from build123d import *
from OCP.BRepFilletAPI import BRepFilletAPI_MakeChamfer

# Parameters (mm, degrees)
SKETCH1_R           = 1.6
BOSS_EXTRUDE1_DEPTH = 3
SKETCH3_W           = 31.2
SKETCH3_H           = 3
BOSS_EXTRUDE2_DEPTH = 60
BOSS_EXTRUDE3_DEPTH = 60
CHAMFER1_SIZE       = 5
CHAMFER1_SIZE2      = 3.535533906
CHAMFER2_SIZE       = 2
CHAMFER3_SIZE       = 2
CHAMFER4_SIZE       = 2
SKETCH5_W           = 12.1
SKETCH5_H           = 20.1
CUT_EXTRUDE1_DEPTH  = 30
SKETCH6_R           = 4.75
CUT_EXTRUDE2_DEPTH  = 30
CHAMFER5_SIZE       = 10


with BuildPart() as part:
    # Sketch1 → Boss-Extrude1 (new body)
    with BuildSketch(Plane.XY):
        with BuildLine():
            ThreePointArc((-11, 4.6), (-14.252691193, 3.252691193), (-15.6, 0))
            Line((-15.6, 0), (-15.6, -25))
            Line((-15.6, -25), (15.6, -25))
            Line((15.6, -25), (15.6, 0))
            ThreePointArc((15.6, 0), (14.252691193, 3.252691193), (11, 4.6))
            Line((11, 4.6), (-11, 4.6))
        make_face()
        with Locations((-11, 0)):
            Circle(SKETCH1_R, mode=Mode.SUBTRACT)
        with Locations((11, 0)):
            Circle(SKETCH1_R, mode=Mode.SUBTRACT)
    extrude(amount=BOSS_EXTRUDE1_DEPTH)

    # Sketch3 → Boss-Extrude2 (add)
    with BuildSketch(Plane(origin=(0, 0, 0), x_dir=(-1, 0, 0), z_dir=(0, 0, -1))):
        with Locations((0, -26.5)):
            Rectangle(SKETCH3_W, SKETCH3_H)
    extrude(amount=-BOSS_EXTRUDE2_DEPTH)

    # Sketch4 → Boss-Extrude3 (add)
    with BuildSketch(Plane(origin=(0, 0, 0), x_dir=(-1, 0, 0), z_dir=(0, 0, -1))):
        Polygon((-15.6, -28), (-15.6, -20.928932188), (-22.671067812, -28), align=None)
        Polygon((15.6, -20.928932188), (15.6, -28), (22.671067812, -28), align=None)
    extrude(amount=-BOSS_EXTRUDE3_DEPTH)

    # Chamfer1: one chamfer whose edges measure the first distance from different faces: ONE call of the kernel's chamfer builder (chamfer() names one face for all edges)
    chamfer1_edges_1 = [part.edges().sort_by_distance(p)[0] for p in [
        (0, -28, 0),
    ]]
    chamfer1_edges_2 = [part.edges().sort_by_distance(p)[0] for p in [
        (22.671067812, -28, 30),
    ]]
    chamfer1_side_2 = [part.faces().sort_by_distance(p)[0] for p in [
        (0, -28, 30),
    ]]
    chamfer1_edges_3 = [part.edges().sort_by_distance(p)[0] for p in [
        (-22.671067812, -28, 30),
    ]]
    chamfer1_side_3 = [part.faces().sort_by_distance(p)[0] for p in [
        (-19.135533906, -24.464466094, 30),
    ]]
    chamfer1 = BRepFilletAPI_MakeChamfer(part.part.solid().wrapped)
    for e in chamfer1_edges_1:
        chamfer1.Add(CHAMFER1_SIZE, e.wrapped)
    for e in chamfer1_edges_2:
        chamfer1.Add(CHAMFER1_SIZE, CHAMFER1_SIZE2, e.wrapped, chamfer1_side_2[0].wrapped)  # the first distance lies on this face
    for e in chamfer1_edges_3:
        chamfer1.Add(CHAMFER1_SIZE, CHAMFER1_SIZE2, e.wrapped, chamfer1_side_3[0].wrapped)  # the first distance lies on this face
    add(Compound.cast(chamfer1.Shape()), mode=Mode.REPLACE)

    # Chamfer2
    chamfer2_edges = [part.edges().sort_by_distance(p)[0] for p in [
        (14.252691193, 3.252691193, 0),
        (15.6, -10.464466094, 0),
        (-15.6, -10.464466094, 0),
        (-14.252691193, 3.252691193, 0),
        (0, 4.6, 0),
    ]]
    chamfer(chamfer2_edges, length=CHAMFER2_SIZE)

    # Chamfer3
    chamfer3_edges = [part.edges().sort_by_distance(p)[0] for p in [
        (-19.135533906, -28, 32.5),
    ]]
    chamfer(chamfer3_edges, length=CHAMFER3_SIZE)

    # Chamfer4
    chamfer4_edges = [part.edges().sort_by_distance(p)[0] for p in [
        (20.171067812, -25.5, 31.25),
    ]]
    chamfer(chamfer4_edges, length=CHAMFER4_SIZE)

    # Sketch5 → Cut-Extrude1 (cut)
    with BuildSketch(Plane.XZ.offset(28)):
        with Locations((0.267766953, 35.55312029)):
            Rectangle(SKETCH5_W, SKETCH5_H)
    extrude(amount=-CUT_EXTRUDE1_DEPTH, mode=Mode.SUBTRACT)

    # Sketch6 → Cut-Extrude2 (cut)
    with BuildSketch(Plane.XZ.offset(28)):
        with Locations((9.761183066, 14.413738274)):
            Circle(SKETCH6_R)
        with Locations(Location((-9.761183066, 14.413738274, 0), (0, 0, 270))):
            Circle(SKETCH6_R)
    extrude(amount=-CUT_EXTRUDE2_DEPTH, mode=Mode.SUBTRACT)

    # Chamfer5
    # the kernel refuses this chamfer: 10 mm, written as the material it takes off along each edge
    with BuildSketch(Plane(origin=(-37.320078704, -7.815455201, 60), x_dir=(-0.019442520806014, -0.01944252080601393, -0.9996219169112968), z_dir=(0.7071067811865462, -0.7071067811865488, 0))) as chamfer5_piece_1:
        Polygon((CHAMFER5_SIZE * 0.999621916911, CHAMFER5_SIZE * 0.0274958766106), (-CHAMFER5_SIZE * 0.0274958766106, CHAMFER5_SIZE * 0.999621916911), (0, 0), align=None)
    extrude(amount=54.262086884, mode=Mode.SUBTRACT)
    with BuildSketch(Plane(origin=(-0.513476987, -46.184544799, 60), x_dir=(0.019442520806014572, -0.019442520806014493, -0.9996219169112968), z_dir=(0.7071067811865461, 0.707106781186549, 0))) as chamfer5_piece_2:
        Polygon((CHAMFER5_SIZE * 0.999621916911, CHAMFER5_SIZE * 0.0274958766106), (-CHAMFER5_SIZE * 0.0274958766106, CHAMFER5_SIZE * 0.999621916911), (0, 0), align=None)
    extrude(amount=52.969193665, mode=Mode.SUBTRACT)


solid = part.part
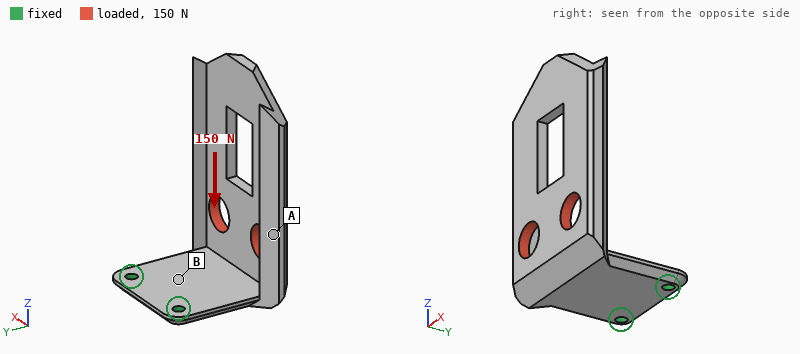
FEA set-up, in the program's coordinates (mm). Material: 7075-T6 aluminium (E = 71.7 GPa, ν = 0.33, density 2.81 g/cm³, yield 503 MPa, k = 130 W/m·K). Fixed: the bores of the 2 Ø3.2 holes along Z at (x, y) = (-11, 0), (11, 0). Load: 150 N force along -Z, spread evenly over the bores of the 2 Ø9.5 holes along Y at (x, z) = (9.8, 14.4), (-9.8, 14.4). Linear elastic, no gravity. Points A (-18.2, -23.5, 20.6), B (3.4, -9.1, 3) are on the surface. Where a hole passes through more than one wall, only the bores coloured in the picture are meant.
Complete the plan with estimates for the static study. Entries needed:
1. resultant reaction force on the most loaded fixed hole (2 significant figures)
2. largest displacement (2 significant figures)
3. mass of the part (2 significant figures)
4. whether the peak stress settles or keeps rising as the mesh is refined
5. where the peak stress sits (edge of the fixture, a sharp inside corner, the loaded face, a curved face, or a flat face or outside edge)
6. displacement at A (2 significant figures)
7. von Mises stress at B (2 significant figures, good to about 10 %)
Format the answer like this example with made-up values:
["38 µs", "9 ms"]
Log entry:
["75 N", "0.76 mm", "23 g", "keeps rising", "edge of the fixture", "0.29 mm", "52 MPa"]
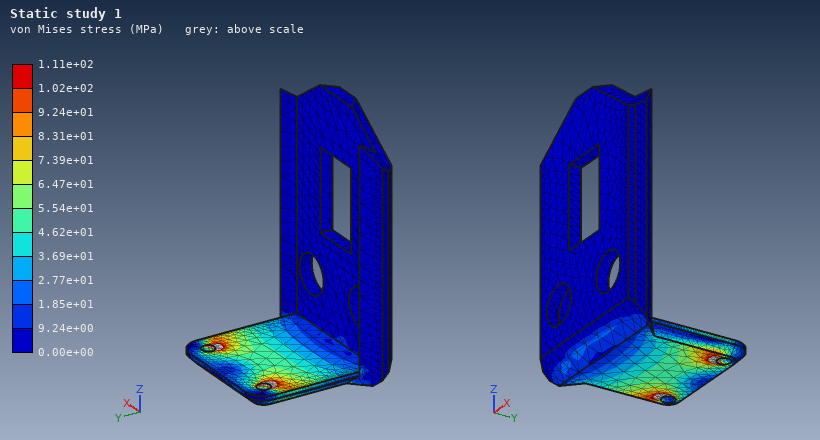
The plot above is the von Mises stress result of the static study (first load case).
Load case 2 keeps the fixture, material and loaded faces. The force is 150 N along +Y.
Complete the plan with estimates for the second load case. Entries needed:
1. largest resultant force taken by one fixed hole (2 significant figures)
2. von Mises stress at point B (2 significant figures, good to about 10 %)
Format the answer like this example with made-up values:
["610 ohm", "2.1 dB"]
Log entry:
["75 N", "41 MPa"]
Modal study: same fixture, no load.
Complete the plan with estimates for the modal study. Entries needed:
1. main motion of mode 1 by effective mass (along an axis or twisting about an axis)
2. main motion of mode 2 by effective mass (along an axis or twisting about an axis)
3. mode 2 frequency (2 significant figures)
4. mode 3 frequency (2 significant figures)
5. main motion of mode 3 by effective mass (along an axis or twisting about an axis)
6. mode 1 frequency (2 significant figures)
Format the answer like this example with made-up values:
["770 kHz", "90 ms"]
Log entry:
["along Y", "along X", "760 Hz", "1600 Hz", "along Z", "400 Hz"]
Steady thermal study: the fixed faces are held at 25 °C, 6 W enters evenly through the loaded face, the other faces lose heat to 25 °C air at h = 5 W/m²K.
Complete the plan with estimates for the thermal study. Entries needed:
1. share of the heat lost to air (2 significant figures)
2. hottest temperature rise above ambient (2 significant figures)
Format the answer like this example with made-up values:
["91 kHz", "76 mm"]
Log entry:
["8.1 %", "20 K"]
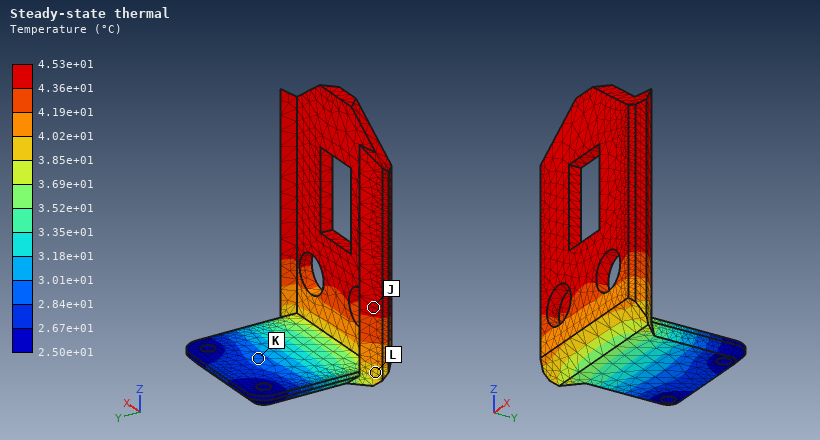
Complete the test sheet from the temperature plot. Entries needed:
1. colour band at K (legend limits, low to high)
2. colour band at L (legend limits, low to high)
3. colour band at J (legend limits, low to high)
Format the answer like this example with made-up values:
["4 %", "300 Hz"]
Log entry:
["2.84e+01 to 3.01e+01 °C", "3.85e+01 to 4.02e+01 °C", "4.36e+01 to 4.53e+01 °C"]
